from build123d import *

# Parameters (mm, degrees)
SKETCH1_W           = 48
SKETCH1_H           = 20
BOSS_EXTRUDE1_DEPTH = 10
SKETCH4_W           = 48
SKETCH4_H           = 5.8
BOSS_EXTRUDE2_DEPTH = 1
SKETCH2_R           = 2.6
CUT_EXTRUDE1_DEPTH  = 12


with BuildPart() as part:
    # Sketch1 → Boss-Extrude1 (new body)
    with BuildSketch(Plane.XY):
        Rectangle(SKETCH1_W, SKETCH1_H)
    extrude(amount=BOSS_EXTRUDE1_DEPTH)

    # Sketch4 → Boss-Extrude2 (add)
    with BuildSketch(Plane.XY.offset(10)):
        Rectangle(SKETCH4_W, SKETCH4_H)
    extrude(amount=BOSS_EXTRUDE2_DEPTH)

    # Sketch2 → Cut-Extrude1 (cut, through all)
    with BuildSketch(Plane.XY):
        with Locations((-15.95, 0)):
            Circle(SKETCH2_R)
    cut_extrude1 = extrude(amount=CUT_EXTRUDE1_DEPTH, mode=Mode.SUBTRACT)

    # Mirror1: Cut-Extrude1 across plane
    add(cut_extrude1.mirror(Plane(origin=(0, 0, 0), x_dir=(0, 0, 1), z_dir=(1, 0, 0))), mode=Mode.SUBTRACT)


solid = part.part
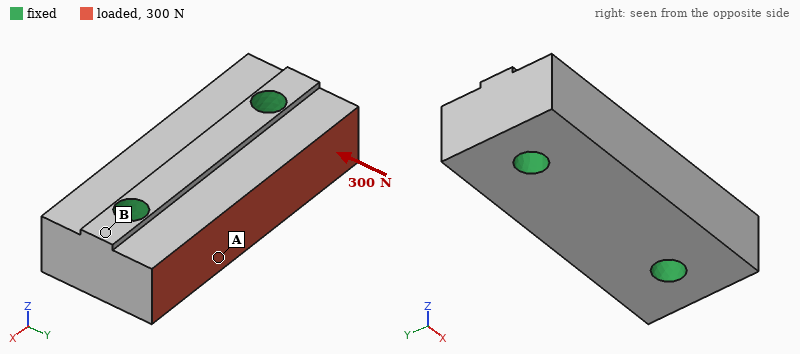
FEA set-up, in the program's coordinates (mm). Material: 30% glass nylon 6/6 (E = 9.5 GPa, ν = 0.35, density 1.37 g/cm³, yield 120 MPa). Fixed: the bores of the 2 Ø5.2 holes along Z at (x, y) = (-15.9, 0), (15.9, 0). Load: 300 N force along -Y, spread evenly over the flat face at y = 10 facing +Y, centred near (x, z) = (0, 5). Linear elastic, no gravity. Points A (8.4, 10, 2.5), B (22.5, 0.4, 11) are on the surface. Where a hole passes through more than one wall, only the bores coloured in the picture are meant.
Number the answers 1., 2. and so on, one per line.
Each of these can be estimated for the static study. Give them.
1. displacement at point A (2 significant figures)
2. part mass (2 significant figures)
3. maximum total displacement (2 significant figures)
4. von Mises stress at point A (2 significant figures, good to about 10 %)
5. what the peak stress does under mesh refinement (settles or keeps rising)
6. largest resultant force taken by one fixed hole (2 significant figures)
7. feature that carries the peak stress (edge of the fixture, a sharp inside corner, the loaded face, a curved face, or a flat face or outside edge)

1. 1.5 µm
2. 13 g
3. 2.0 µm
4. 0.55 MPa
5. keeps rising
6. 150 N
7. edge of the fixture
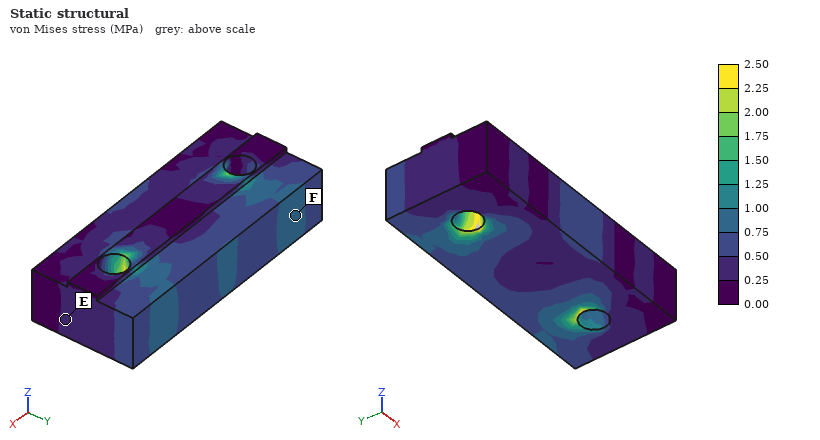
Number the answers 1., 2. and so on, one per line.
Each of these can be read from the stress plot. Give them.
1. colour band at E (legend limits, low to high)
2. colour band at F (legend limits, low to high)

1. 0.25 to 0.50 MPa
2. 0.75 to 1.00 MPa
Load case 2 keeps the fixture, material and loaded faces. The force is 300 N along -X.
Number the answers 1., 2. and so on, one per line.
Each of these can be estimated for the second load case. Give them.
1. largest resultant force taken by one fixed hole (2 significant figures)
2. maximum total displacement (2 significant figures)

1. 170 N
2. 3.9 µm
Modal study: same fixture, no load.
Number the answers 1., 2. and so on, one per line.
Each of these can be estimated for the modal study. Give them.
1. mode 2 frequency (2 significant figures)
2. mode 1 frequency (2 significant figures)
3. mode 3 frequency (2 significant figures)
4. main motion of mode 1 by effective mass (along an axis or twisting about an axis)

1. 19 kHz
2. 18 kHz
3. 19 kHz
4. along Z
